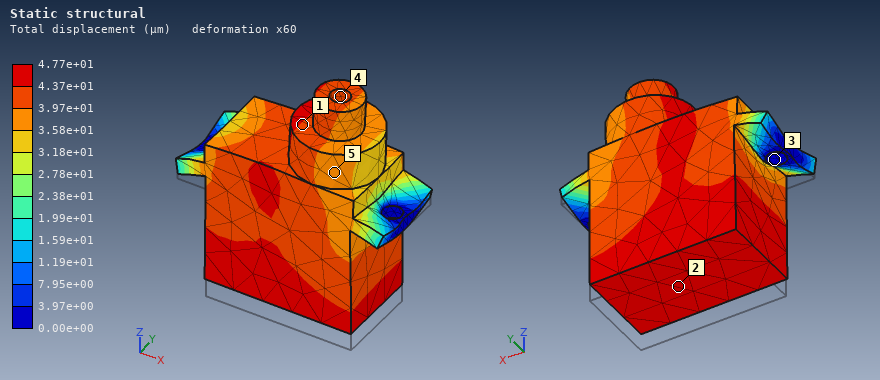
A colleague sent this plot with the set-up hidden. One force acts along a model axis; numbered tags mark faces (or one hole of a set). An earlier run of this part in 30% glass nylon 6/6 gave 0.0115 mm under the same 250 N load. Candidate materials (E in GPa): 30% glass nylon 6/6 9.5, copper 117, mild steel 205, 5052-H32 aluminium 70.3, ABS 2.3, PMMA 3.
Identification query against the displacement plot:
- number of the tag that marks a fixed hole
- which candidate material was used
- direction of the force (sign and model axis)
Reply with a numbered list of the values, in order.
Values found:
1. 3
2. ABS
3. +Z
